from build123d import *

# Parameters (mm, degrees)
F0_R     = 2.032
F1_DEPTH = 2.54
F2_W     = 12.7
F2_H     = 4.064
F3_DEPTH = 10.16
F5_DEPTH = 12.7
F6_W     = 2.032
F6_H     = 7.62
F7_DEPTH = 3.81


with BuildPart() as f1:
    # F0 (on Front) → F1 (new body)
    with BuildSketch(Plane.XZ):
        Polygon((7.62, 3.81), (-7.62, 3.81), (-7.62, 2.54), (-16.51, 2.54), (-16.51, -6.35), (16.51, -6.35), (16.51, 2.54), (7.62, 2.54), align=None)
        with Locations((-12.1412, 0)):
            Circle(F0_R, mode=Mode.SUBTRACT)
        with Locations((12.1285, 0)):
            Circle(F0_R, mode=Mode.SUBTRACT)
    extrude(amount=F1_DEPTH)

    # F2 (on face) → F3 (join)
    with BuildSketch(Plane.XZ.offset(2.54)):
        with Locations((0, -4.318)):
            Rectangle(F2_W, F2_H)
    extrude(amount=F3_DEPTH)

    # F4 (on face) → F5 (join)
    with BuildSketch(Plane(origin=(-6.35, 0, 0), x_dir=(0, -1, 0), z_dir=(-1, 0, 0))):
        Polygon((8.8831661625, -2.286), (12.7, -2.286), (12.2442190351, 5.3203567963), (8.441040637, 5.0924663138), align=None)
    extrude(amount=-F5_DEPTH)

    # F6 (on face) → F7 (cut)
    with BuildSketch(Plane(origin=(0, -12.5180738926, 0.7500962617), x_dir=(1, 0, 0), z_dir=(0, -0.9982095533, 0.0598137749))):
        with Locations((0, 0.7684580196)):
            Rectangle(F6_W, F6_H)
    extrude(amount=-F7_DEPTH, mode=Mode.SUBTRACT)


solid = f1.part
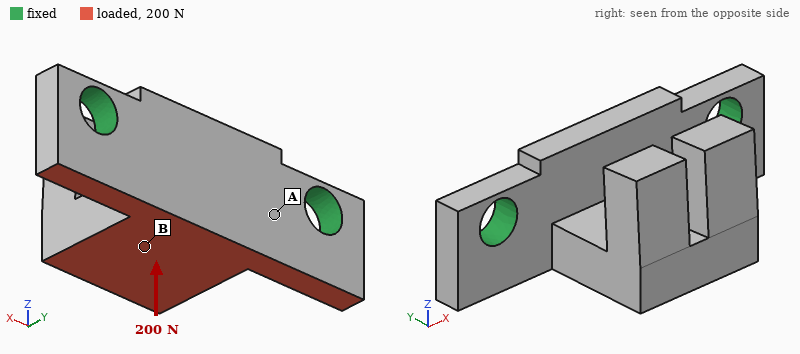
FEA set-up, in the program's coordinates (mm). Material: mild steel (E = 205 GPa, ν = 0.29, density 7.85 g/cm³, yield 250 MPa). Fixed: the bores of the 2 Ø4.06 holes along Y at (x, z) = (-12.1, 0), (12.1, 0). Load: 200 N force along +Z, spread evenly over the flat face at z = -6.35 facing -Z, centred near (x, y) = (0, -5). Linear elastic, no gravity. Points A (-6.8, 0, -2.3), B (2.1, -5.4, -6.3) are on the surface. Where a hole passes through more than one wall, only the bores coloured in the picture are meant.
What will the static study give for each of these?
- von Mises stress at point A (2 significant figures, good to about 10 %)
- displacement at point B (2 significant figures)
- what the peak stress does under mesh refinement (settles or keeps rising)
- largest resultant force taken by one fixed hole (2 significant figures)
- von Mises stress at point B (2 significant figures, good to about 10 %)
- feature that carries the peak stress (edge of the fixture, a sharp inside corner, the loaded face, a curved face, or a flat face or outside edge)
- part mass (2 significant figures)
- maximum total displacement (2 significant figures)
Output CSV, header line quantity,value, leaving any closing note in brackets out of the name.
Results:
quantity,value
von Mises stress at point A,23 MPa
displacement at point B,5.1 µm
what the peak stress does under mesh refinement,keeps rising
largest resultant force taken by one fixed hole,100 N
von Mises stress at point B,8.0 MPa
feature that carries the peak stress,edge of the fixture
part mass,12 g
maximum total displacement,12 µm
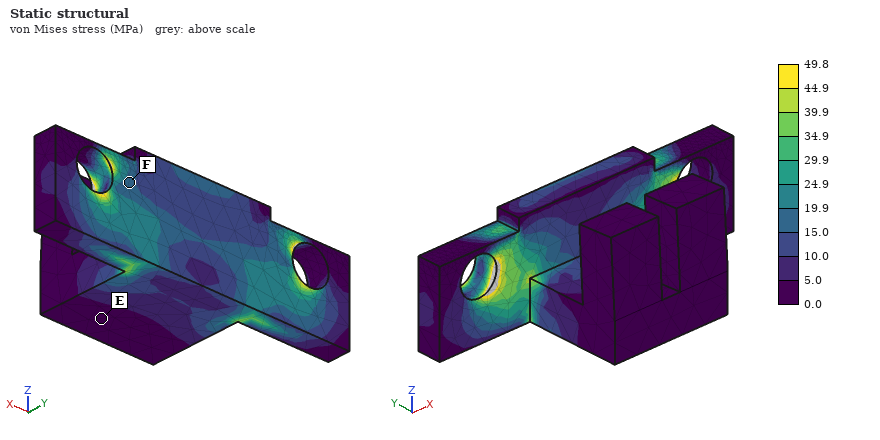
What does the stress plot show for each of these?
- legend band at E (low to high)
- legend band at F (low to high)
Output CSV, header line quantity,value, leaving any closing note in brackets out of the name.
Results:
quantity,value
legend band at E,0.0 to 5.0 MPa
legend band at F,15.0 to 19.9 MPa
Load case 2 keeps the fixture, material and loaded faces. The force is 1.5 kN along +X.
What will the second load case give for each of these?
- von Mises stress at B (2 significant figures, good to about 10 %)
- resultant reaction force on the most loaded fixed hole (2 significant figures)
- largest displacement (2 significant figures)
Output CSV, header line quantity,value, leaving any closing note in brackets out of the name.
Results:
quantity,value
von Mises stress at B,45 MPa
resultant reaction force on the most loaded fixed hole,880 N
largest displacement,13 µm
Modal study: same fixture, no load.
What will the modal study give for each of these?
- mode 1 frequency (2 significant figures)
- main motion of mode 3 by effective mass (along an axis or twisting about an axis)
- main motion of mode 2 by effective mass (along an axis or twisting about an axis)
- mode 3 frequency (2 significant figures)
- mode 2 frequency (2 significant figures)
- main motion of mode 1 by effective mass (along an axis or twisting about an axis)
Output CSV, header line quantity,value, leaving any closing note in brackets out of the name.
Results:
quantity,value
mode 1 frequency,6700 Hz
main motion of mode 3 by effective mass,along Y
main motion of mode 2 by effective mass,along X
mode 3 frequency,16 kHz
mode 2 frequency,14 kHz
main motion of mode 1 by effective mass,along Z
